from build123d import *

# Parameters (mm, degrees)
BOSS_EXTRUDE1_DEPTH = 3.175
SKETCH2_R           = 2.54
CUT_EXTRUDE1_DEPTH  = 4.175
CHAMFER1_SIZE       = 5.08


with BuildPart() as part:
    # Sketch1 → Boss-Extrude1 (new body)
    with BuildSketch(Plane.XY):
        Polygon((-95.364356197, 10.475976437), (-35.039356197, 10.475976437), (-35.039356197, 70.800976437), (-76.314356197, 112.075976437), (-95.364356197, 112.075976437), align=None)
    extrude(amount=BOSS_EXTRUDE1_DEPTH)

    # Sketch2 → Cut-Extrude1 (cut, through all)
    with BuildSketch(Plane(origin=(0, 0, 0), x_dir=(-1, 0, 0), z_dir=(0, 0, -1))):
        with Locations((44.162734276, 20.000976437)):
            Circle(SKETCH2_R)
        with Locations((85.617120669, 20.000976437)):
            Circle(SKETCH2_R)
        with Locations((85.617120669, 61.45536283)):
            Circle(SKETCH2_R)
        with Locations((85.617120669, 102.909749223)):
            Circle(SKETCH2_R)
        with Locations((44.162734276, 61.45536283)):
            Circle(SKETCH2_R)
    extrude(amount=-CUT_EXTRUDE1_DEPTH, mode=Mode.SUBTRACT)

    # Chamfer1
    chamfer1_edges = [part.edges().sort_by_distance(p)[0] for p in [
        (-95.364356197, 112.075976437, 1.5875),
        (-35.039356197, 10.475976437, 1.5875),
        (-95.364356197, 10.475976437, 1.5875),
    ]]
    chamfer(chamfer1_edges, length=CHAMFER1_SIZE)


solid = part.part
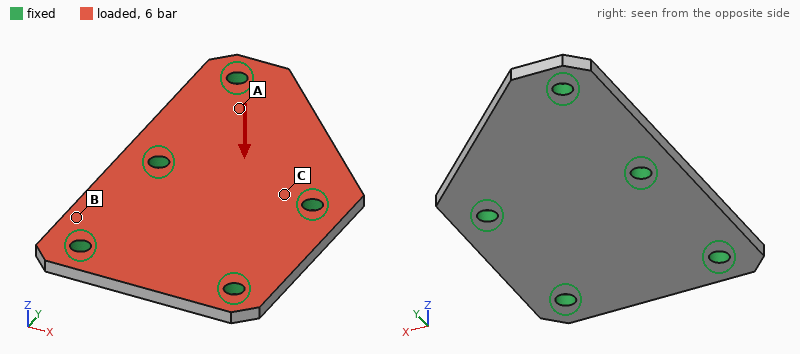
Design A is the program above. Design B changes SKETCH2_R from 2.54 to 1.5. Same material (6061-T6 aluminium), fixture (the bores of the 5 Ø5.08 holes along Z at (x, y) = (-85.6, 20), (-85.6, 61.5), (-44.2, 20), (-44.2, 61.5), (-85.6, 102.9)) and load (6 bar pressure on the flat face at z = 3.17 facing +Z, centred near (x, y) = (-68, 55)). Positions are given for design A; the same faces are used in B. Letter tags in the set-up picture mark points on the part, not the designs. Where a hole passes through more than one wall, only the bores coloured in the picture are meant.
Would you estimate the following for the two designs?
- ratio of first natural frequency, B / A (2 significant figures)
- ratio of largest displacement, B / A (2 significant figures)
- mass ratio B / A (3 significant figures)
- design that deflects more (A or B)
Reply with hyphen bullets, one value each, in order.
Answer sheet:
- 0.89
- 1.2
- 1.01
- B
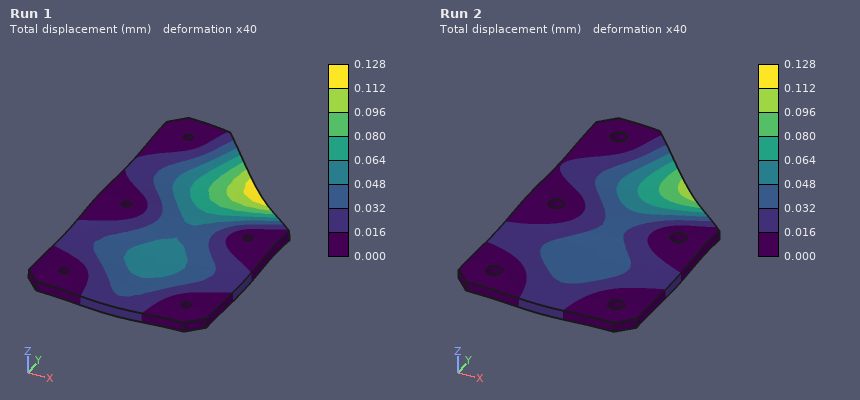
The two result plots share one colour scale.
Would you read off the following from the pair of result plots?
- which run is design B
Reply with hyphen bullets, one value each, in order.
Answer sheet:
- Run 1
